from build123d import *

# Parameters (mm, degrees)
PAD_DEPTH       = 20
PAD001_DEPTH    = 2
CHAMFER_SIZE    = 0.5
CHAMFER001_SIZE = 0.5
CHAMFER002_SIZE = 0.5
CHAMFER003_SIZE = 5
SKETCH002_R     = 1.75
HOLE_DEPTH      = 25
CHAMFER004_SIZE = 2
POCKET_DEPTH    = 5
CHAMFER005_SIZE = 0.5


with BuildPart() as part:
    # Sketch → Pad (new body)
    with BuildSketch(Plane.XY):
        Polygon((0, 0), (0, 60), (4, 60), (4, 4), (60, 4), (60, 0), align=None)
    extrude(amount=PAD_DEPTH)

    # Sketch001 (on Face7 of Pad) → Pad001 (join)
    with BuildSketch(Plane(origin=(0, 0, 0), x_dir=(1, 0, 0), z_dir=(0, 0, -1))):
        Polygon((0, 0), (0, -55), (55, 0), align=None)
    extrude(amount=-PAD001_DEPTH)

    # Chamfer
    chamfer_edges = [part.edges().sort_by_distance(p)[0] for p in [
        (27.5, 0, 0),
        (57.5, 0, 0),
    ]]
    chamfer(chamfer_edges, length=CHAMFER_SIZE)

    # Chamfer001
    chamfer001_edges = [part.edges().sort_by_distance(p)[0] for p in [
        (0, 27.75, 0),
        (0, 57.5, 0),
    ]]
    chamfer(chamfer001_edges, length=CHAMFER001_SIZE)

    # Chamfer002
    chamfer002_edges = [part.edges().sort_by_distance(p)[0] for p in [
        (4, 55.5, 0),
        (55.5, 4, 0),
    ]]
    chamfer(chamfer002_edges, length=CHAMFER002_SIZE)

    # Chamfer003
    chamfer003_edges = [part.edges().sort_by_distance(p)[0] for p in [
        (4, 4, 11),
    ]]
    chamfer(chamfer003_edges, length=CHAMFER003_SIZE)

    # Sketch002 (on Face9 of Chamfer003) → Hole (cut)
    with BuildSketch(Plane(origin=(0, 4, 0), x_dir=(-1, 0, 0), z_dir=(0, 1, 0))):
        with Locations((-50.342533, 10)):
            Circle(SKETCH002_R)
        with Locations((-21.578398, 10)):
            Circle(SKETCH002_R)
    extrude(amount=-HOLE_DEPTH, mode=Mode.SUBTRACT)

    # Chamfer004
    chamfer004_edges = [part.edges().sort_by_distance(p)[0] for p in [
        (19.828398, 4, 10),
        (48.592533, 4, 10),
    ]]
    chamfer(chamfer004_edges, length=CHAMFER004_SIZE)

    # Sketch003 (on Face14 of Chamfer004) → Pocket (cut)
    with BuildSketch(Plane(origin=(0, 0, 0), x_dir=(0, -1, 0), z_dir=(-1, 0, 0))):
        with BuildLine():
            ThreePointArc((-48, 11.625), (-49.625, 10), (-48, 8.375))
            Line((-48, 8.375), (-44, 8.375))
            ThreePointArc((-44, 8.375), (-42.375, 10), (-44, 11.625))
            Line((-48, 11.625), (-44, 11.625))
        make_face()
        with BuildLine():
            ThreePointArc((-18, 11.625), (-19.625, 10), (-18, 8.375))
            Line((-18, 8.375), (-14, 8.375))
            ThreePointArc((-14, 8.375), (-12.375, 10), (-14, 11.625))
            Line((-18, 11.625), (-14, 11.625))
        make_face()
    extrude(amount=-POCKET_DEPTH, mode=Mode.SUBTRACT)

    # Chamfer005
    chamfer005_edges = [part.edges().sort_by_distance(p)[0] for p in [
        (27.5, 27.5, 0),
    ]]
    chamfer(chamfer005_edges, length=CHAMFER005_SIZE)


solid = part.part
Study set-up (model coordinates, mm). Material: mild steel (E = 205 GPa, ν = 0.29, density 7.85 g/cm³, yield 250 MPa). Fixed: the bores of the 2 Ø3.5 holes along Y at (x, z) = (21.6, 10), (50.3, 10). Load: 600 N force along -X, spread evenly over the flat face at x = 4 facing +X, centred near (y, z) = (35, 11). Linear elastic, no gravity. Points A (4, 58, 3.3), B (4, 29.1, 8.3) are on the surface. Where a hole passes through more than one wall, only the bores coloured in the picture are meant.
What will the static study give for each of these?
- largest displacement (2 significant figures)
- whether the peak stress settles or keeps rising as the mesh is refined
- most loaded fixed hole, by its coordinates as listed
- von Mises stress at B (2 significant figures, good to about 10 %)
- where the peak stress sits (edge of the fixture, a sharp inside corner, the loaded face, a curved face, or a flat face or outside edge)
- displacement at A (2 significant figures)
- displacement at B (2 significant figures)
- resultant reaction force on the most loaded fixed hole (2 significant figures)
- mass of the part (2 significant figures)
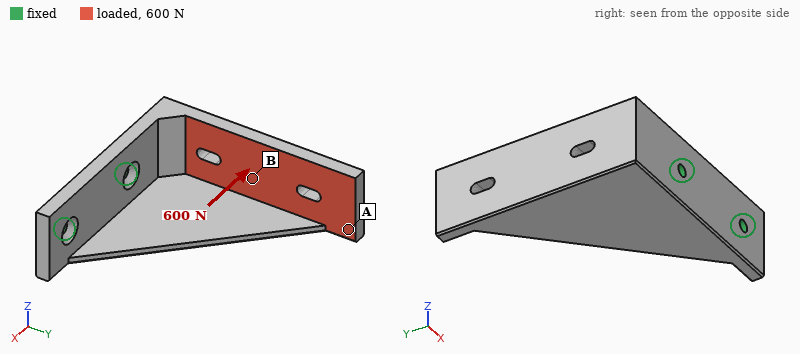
0.22 mm
keeps rising
(50.3, 10)
58 MPa
edge of the fixture
0.13 mm
0.074 mm
950 N
89 g
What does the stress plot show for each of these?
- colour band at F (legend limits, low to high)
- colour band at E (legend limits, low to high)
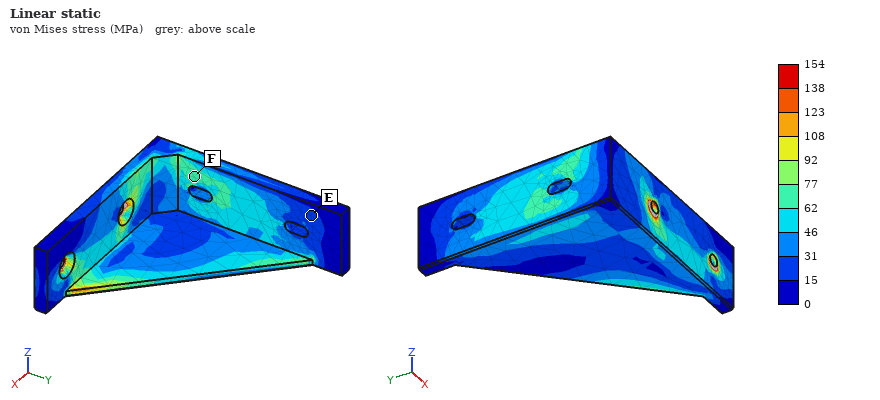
62 to 77 MPa
15 to 31 MPa
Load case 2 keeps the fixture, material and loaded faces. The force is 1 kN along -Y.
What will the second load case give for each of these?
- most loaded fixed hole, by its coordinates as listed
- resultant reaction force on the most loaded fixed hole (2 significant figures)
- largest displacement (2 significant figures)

(21.6, 10)
1.6 kN
0.10 mm
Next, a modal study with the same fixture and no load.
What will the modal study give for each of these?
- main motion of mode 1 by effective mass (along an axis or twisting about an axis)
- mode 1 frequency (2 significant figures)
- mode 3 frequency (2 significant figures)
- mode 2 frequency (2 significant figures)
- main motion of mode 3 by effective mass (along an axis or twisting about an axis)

along Z
990 Hz
4200 Hz
2000 Hz
along Y
